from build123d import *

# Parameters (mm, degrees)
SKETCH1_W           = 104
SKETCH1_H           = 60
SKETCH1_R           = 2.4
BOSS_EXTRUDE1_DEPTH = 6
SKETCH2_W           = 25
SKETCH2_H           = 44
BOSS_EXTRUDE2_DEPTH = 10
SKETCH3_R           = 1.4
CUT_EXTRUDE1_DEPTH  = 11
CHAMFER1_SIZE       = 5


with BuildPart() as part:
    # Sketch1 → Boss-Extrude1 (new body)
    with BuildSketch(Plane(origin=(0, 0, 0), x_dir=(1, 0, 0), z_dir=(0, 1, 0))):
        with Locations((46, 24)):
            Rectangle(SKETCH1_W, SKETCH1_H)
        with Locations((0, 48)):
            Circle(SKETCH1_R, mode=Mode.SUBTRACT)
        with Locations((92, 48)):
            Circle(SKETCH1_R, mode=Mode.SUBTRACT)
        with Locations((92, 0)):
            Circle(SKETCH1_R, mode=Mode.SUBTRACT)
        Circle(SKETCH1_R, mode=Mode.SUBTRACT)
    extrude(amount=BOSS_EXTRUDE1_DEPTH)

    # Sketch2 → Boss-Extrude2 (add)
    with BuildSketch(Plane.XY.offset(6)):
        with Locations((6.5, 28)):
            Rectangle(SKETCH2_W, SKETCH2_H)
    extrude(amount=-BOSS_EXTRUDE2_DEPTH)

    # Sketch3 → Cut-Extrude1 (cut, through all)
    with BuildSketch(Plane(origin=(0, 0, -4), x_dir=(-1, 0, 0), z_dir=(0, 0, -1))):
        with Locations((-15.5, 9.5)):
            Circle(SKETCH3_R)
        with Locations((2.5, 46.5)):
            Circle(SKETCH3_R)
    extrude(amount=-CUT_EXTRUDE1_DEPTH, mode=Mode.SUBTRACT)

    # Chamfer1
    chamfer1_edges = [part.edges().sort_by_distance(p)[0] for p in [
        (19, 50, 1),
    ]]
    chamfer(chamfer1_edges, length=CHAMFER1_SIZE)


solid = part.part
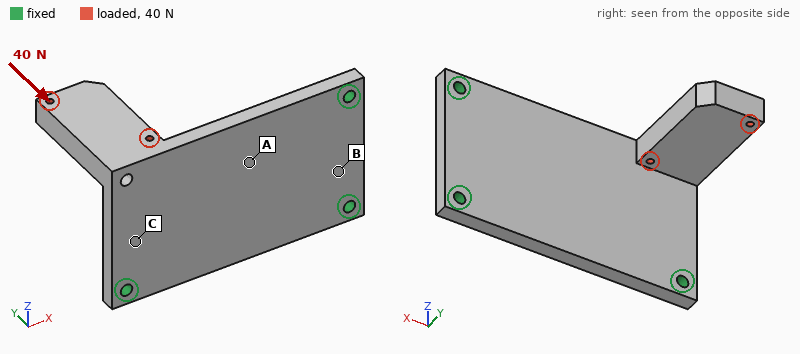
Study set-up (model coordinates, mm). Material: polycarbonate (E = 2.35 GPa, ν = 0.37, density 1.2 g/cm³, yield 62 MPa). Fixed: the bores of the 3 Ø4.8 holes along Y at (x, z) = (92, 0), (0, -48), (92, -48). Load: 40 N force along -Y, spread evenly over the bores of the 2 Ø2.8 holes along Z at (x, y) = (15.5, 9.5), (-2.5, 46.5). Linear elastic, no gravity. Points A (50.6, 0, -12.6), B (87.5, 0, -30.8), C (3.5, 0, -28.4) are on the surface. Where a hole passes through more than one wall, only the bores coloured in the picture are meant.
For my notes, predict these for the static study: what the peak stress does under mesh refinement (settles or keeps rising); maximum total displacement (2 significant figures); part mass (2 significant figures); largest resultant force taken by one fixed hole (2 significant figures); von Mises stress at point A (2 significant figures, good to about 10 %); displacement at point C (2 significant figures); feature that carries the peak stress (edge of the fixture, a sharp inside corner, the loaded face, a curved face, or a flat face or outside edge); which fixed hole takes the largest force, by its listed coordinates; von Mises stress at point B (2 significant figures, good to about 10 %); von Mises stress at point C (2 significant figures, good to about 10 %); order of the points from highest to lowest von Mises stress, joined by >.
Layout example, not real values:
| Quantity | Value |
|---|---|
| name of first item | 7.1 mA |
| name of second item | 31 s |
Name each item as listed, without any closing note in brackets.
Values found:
| Quantity | Value |
|---|---|
| what the peak stress does under mesh refinement | keeps rising |
| maximum total displacement | 1.3 mm |
| part mass | 57 g |
| largest resultant force taken by one fixed hole | 34 N |
| von Mises stress at point A | 2.2 MPa |
| displacement at point C | 0.19 mm |
| feature that carries the peak stress | edge of the fixture |
| which fixed hole takes the largest force, by its listed coordinates | (0, -48) |
| von Mises stress at point B | 0.81 MPa |
| von Mises stress at point C | 3.4 MPa |
| order of the points from highest to lowest von Mises stress, joined by > | C > A > B |
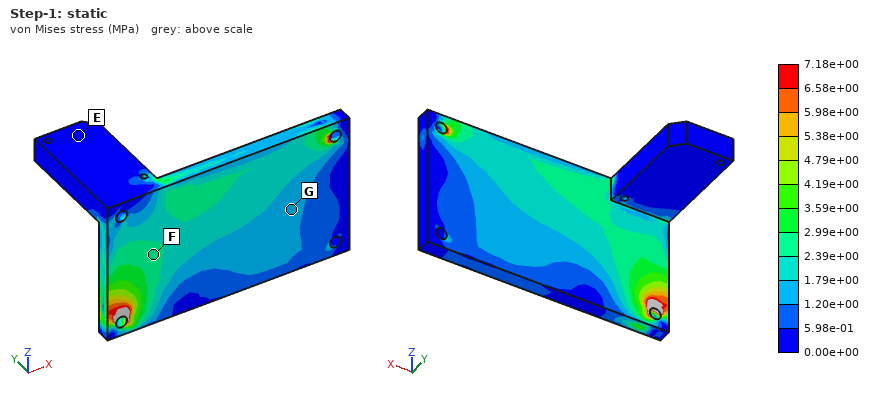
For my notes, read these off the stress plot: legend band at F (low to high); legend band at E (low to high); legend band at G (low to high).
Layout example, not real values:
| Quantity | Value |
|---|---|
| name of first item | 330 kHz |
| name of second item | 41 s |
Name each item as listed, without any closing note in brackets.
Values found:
| Quantity | Value |
|---|---|
| legend band at F | 2.39e+00 to 2.99e+00 MPa |
| legend band at E | 0.00e+00 to 5.98e-01 MPa |
| legend band at G | 1.20e+00 to 1.79e+00 MPa |
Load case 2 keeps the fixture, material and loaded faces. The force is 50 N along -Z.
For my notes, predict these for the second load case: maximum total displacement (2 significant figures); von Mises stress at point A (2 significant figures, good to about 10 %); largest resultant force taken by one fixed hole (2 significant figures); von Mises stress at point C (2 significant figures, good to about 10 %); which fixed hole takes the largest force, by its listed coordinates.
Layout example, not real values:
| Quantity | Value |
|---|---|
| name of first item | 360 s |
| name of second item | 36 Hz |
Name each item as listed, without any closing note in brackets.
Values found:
| Quantity | Value |
|---|---|
| maximum total displacement | 1.5 mm |
| von Mises stress at point A | 2.2 MPa |
| largest resultant force taken by one fixed hole | 43 N |
| von Mises stress at point C | 2.7 MPa |
| which fixed hole takes the largest force, by its listed coordinates | (0, -48) |
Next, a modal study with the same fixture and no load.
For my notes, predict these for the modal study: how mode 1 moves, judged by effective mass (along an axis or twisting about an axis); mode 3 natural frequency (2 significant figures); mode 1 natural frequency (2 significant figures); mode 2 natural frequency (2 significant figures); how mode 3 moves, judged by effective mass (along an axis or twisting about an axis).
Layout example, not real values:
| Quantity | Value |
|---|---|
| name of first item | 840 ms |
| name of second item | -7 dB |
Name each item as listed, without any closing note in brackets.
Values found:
| Quantity | Value |
|---|---|
| how mode 1 moves, judged by effective mass | along Y |
| mode 3 natural frequency | 600 Hz |
| mode 1 natural frequency | 230 Hz |
| mode 2 natural frequency | 450 Hz |
| how mode 3 moves, judged by effective mass | along Y |
